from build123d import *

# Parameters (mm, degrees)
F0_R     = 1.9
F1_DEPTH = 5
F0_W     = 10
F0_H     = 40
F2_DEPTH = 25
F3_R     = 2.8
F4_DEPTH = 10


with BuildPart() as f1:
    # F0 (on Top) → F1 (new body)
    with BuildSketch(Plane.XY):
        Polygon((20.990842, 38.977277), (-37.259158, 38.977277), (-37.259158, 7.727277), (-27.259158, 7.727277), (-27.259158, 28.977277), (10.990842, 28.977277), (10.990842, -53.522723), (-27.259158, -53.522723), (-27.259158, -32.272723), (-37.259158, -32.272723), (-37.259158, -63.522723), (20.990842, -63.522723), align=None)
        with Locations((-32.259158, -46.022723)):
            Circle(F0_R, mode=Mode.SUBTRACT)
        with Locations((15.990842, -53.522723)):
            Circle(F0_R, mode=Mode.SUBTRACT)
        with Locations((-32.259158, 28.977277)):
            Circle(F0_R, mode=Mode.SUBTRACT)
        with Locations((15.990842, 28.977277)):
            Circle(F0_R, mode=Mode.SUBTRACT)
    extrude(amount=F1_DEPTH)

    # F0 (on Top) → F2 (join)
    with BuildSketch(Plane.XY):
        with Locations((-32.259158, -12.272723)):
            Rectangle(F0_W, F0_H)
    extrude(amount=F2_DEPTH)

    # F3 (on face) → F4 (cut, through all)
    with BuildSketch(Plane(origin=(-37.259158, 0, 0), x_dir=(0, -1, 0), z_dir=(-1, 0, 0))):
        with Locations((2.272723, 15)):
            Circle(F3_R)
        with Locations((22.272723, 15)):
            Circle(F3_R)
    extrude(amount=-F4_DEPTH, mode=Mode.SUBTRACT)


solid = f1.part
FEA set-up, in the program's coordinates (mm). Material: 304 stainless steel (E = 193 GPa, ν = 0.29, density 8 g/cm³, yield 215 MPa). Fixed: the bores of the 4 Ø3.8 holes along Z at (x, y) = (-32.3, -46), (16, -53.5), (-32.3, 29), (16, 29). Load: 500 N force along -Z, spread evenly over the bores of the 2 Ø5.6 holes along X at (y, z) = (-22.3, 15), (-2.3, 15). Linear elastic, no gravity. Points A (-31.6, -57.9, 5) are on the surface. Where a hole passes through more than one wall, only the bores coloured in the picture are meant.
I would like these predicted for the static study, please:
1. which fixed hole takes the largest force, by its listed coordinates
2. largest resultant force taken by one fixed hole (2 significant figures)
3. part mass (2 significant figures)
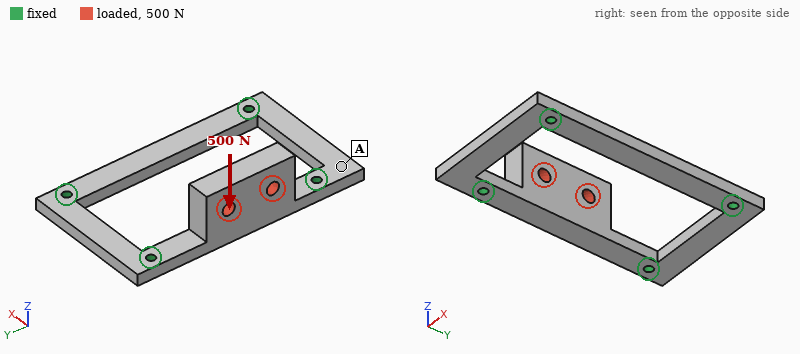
(-32.3, -46)
320 N
170 g
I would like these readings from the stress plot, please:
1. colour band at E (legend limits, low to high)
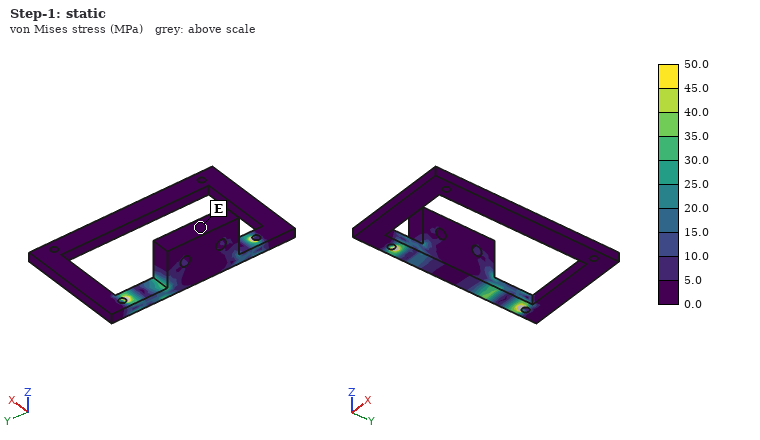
0.0 to 5.0 MPa
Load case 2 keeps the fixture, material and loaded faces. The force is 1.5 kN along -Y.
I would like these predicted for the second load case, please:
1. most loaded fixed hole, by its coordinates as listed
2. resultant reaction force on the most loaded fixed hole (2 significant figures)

(-32.3, -46)
880 N
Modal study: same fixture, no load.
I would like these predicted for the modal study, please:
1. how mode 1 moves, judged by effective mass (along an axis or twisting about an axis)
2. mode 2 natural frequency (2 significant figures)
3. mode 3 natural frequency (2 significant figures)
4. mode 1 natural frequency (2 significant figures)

along X
3800 Hz
3900 Hz
2100 Hz
